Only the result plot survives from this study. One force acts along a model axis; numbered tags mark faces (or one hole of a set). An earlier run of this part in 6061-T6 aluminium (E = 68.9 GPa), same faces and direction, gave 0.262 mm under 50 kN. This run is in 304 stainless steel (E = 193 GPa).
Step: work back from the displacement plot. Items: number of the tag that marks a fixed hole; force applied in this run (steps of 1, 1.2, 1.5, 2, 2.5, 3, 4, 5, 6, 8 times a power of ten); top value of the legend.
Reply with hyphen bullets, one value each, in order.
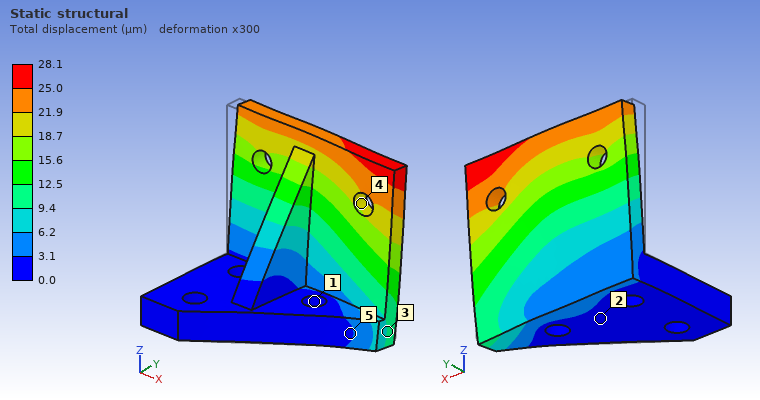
- 1
- 15 kN
- 28.1 µm
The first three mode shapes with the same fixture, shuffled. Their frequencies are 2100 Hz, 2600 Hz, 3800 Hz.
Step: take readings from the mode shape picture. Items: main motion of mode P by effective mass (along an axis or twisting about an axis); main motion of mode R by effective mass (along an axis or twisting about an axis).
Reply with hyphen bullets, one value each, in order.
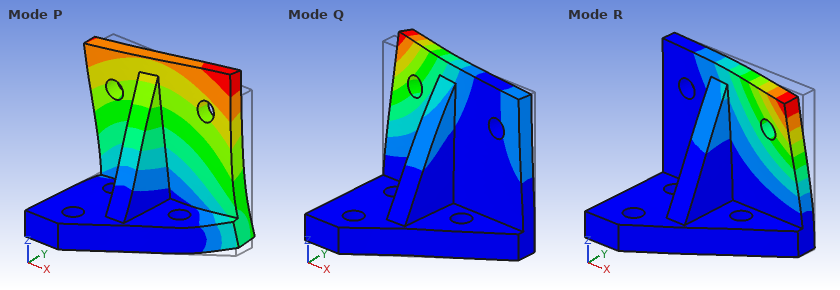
- along X
- along Y
